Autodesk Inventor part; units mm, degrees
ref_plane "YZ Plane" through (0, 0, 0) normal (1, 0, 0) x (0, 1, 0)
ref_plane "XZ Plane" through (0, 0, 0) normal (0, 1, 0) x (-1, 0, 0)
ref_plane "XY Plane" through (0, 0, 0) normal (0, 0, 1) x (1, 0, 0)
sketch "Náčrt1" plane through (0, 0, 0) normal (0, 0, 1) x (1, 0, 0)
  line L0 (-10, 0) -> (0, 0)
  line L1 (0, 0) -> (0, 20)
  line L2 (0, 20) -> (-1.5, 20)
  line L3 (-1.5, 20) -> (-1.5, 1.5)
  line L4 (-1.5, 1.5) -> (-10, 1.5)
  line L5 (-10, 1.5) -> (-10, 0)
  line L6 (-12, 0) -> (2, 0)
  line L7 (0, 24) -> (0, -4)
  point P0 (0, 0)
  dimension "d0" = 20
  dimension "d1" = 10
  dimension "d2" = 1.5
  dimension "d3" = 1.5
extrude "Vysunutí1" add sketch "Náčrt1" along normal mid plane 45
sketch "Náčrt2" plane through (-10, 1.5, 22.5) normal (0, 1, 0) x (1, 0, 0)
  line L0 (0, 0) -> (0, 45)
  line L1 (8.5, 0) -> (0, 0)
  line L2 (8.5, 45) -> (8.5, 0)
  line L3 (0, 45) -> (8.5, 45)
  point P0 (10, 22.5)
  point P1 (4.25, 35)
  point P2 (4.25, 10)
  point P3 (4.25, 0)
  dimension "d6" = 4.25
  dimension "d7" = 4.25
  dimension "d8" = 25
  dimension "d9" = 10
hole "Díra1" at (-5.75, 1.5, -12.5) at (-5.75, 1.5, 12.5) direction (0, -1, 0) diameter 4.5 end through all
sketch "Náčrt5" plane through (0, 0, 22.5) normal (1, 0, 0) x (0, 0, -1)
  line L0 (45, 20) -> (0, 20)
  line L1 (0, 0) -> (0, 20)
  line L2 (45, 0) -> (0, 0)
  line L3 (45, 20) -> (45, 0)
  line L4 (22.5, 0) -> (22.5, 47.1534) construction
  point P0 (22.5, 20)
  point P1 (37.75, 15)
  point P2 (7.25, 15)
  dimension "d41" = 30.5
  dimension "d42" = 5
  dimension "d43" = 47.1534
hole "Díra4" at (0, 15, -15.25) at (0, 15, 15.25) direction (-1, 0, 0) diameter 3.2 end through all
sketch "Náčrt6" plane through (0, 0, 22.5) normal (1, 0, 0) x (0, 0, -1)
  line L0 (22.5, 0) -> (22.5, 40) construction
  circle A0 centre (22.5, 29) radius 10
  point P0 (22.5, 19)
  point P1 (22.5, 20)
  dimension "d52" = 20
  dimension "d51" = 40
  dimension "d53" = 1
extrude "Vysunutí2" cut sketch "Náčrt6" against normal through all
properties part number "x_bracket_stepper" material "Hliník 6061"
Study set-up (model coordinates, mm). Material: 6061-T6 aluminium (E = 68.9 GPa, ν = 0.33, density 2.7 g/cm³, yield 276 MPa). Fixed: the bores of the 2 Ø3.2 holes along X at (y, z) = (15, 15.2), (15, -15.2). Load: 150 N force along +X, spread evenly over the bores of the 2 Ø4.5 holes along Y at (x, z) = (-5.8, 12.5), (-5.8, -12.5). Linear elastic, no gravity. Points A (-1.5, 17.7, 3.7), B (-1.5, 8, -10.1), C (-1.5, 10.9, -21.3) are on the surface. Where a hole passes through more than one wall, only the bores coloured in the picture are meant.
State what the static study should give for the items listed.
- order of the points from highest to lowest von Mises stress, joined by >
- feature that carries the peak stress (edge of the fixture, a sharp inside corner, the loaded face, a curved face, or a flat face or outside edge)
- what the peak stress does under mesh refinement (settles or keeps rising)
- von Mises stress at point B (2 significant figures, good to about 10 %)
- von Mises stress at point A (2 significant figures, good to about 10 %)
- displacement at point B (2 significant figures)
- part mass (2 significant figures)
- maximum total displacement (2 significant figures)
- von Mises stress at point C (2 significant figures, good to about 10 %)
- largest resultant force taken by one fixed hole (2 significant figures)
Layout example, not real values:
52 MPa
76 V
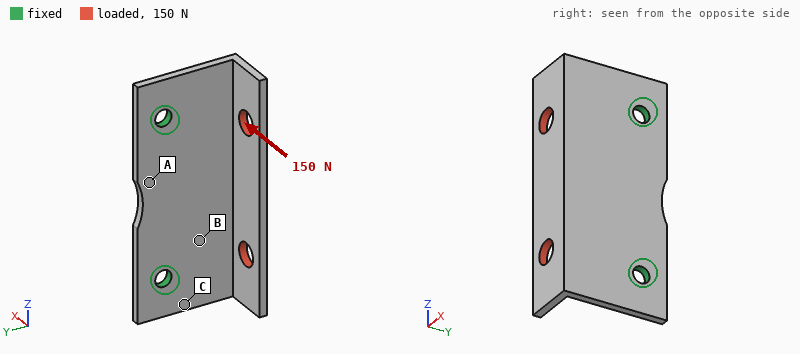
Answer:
C > B > A
edge of the fixture
keeps rising
59 MPa
27 MPa
0.066 mm
5.0 g
0.27 mm
98 MPa
75 N
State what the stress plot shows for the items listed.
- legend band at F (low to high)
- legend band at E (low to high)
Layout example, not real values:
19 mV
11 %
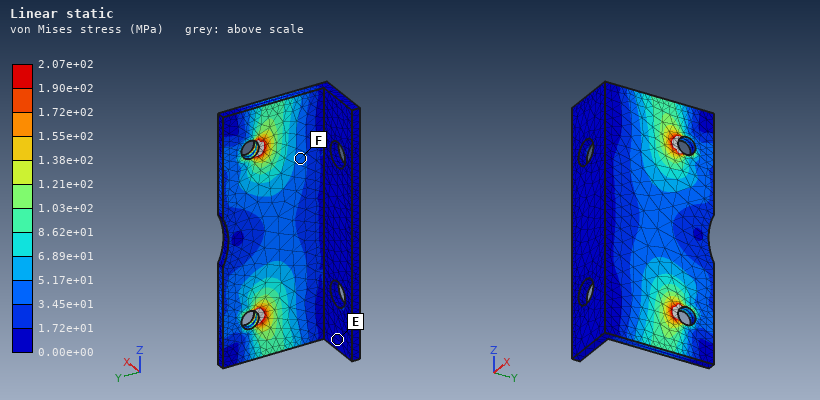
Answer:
3.45e+01 to 5.17e+01 MPa
0.00e+00 to 1.72e+01 MPa
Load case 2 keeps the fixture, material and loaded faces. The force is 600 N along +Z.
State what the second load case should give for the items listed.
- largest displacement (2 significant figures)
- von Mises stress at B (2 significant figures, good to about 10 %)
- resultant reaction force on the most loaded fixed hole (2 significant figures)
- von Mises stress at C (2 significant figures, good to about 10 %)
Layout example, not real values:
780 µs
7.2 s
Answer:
0.25 mm
78 MPa
400 N
81 MPa
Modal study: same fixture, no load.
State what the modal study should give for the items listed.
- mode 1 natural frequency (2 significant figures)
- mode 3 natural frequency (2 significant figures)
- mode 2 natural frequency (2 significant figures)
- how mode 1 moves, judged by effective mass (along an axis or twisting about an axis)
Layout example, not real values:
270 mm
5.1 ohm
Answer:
2700 Hz
8800 Hz
4300 Hz
along X
